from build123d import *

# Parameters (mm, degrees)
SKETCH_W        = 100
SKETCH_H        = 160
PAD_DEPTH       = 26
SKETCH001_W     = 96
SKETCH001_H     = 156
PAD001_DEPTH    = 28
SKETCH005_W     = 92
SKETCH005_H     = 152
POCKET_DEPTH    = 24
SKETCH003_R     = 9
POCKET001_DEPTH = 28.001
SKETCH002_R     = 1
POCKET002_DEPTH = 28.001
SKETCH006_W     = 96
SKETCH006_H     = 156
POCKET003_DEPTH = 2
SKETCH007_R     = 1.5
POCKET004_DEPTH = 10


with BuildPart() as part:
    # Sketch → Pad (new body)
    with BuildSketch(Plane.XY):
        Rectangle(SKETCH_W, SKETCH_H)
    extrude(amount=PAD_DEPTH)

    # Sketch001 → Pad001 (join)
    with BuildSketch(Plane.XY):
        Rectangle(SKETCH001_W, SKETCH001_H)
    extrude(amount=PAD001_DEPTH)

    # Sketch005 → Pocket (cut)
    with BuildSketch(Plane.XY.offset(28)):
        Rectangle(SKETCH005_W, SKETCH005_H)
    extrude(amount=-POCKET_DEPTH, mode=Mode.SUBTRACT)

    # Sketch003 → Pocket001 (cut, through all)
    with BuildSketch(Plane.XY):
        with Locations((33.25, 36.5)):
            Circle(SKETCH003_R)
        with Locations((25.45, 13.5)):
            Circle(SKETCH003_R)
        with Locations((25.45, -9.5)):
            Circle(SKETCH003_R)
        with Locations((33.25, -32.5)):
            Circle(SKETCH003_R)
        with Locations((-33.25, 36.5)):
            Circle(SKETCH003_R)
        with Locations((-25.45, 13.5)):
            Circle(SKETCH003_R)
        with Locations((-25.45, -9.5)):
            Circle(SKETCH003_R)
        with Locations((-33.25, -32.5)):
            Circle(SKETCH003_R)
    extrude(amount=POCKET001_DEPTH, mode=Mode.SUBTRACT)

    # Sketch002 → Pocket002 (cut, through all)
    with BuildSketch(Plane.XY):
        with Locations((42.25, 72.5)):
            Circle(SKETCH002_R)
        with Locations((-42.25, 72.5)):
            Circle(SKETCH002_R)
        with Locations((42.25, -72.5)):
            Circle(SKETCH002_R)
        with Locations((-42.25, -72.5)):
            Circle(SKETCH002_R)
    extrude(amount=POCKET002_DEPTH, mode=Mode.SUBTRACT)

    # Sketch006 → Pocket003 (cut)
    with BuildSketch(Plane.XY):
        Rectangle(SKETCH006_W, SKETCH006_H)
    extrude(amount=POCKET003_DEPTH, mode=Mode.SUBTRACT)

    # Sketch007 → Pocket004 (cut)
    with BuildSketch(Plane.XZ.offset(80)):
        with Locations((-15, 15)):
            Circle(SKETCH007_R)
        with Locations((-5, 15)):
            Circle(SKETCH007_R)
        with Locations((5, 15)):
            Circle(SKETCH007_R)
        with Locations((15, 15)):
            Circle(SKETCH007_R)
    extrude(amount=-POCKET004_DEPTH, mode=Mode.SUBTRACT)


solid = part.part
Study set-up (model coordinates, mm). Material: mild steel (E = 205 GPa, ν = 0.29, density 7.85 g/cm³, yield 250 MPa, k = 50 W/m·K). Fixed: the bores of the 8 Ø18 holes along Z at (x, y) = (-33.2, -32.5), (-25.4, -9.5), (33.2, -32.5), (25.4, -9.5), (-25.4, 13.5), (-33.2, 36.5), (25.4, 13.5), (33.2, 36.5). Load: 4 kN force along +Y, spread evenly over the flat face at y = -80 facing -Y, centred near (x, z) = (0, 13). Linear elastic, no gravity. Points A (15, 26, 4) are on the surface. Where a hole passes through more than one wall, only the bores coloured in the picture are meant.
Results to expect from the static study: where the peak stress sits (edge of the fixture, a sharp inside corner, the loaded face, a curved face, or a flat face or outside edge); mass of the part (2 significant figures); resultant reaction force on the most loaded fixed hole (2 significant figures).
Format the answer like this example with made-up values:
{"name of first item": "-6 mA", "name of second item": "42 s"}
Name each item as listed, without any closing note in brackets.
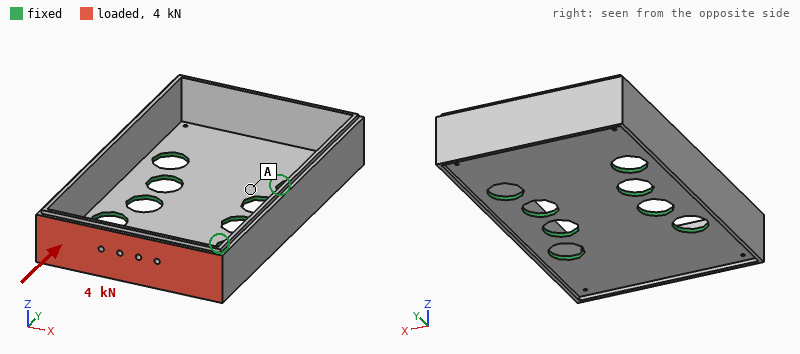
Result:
{"where the peak stress sits": "a flat face or outside edge", "mass of the part": "600 g", "resultant reaction force on the most loaded fixed hole": "1.2 kN"}
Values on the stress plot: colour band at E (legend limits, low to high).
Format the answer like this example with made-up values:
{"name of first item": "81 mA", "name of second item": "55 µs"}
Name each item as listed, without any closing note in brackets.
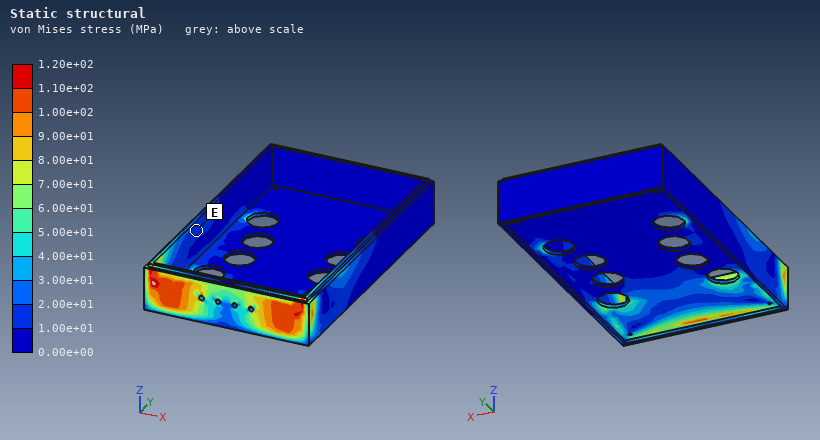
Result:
{"colour band at E": "1.00e+01 to 2.00e+01 MPa"}
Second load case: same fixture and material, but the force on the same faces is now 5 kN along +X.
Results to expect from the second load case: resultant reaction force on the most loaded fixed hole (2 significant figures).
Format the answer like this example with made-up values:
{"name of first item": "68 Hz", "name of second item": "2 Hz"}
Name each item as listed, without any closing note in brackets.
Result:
{"resultant reaction force on the most loaded fixed hole": "4.0 kN"}
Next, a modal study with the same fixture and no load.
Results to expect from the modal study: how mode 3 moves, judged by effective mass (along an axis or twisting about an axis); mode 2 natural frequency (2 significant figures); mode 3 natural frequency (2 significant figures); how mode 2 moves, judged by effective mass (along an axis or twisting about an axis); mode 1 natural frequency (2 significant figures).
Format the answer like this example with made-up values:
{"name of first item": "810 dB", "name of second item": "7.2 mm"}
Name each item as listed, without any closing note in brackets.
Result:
{"how mode 3 moves, judged by effective mass": "along Z", "mode 2 natural frequency": "2300 Hz", "mode 3 natural frequency": "2400 Hz", "how mode 2 moves, judged by effective mass": "along X", "mode 1 natural frequency": "2100 Hz"}
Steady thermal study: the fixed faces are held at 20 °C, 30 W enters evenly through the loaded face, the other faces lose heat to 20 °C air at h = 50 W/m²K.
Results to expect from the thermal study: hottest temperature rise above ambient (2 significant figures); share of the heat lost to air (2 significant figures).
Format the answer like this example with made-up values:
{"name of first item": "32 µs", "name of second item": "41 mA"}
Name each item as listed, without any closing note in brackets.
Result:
{"hottest temperature rise above ambient": "49 K", "share of the heat lost to air": "66 %"}
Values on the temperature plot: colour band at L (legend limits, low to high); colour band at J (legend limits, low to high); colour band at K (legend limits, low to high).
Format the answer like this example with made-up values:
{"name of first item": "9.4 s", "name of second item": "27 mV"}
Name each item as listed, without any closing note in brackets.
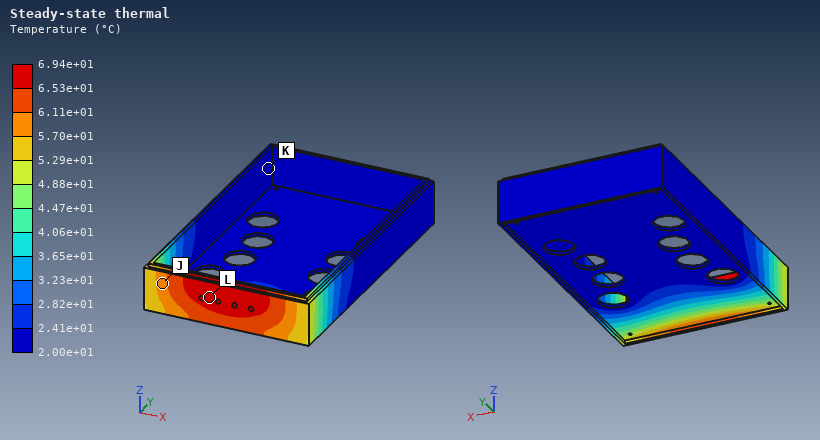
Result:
{"colour band at L": "6.53e+01 to 6.94e+01 °C", "colour band at J": "5.70e+01 to 6.11e+01 °C", "colour band at K": "2.00e+01 to 2.41e+01 °C"}
